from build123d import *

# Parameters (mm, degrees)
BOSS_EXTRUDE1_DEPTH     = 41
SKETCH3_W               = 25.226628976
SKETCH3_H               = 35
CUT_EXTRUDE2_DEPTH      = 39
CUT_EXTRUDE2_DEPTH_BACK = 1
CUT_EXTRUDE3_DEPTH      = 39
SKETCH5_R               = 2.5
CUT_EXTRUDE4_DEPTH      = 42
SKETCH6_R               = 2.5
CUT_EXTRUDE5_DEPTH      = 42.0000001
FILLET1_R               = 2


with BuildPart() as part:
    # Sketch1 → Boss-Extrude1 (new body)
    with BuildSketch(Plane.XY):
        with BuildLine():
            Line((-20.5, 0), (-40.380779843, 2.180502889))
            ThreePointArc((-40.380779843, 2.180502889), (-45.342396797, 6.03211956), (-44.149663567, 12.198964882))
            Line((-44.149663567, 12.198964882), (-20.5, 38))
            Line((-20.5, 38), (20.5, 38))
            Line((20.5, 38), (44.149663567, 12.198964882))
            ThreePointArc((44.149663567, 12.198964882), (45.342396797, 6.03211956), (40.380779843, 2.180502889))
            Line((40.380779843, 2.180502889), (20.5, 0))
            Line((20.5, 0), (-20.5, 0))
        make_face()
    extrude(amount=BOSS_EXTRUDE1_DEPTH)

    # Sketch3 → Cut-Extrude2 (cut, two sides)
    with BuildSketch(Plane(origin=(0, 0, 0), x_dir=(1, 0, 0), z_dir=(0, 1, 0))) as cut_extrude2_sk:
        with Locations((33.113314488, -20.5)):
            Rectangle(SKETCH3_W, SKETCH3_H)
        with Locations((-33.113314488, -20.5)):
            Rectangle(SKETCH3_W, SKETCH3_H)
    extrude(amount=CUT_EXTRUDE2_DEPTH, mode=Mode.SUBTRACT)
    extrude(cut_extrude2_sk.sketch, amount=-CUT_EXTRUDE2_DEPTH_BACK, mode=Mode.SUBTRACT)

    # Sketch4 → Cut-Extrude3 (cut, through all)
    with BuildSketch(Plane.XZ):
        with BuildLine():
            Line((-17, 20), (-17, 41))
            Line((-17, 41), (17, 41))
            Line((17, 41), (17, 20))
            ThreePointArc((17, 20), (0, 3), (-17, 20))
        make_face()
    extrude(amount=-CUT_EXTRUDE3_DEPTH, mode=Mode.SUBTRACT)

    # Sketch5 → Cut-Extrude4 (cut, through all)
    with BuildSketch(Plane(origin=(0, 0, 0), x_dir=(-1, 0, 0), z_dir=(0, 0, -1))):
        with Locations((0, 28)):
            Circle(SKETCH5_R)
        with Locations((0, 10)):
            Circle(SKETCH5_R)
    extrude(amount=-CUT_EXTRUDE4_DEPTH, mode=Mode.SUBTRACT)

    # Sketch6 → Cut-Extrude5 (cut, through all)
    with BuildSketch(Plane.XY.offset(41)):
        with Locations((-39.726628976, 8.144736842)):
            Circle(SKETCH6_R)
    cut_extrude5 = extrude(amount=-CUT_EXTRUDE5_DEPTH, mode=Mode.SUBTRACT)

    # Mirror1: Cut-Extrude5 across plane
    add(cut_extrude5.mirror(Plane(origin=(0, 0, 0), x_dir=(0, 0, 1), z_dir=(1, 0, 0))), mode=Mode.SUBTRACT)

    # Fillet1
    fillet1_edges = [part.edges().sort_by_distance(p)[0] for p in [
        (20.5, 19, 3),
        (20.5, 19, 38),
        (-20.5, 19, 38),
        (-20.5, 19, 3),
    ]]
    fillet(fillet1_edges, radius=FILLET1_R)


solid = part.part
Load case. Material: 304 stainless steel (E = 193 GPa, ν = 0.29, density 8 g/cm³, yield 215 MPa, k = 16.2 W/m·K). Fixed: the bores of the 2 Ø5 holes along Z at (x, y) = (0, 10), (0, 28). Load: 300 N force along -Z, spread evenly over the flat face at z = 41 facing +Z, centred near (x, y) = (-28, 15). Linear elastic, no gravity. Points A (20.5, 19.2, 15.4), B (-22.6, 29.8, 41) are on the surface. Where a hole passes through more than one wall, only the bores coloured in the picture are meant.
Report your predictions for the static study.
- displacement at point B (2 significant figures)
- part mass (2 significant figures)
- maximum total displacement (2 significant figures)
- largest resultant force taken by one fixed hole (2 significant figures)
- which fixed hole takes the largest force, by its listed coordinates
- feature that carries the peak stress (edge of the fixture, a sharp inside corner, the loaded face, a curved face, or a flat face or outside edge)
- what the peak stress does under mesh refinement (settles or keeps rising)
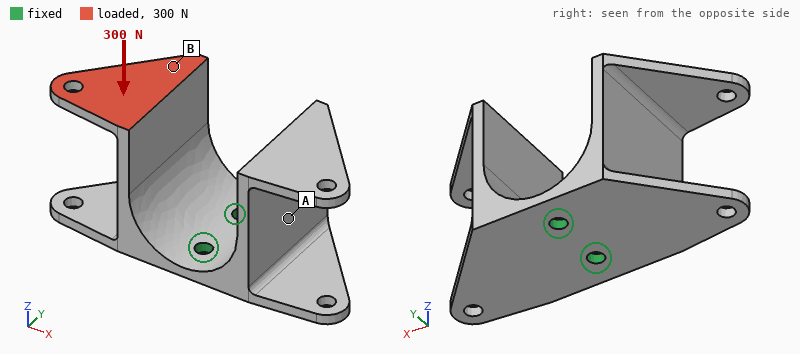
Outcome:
0.12 mm
210 g
0.22 mm
200 N
(0, 10)
edge of the fixture
keeps rising
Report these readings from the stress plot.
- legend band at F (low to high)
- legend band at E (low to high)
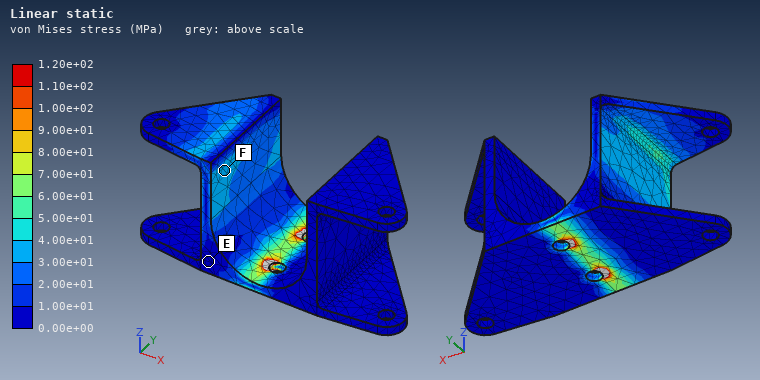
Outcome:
3.00e+01 to 4.00e+01 MPa
0.00e+00 to 1.00e+01 MPa
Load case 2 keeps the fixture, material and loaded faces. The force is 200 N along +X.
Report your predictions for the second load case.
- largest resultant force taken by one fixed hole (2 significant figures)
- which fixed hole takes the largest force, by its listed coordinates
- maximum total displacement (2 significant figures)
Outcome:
140 N
(0, 10)
0.23 mm
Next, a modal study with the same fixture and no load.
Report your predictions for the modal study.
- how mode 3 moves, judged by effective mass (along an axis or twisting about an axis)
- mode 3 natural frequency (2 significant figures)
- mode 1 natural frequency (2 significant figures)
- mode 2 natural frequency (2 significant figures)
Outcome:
twisting about Z
3000 Hz
980 Hz
1000 Hz
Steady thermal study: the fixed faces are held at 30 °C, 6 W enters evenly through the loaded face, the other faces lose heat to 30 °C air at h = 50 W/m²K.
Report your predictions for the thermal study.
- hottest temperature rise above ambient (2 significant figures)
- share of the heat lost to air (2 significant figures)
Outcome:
58 K
85 %
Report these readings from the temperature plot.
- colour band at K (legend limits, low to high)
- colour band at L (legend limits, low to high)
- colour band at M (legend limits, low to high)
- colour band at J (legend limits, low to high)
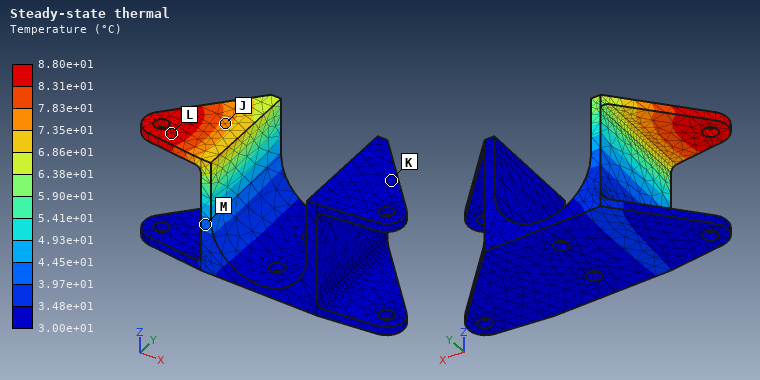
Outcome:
3.00e+01 to 3.48e+01 °C
8.31e+01 to 8.80e+01 °C
3.97e+01 to 4.45e+01 °C
7.35e+01 to 7.83e+01 °C
